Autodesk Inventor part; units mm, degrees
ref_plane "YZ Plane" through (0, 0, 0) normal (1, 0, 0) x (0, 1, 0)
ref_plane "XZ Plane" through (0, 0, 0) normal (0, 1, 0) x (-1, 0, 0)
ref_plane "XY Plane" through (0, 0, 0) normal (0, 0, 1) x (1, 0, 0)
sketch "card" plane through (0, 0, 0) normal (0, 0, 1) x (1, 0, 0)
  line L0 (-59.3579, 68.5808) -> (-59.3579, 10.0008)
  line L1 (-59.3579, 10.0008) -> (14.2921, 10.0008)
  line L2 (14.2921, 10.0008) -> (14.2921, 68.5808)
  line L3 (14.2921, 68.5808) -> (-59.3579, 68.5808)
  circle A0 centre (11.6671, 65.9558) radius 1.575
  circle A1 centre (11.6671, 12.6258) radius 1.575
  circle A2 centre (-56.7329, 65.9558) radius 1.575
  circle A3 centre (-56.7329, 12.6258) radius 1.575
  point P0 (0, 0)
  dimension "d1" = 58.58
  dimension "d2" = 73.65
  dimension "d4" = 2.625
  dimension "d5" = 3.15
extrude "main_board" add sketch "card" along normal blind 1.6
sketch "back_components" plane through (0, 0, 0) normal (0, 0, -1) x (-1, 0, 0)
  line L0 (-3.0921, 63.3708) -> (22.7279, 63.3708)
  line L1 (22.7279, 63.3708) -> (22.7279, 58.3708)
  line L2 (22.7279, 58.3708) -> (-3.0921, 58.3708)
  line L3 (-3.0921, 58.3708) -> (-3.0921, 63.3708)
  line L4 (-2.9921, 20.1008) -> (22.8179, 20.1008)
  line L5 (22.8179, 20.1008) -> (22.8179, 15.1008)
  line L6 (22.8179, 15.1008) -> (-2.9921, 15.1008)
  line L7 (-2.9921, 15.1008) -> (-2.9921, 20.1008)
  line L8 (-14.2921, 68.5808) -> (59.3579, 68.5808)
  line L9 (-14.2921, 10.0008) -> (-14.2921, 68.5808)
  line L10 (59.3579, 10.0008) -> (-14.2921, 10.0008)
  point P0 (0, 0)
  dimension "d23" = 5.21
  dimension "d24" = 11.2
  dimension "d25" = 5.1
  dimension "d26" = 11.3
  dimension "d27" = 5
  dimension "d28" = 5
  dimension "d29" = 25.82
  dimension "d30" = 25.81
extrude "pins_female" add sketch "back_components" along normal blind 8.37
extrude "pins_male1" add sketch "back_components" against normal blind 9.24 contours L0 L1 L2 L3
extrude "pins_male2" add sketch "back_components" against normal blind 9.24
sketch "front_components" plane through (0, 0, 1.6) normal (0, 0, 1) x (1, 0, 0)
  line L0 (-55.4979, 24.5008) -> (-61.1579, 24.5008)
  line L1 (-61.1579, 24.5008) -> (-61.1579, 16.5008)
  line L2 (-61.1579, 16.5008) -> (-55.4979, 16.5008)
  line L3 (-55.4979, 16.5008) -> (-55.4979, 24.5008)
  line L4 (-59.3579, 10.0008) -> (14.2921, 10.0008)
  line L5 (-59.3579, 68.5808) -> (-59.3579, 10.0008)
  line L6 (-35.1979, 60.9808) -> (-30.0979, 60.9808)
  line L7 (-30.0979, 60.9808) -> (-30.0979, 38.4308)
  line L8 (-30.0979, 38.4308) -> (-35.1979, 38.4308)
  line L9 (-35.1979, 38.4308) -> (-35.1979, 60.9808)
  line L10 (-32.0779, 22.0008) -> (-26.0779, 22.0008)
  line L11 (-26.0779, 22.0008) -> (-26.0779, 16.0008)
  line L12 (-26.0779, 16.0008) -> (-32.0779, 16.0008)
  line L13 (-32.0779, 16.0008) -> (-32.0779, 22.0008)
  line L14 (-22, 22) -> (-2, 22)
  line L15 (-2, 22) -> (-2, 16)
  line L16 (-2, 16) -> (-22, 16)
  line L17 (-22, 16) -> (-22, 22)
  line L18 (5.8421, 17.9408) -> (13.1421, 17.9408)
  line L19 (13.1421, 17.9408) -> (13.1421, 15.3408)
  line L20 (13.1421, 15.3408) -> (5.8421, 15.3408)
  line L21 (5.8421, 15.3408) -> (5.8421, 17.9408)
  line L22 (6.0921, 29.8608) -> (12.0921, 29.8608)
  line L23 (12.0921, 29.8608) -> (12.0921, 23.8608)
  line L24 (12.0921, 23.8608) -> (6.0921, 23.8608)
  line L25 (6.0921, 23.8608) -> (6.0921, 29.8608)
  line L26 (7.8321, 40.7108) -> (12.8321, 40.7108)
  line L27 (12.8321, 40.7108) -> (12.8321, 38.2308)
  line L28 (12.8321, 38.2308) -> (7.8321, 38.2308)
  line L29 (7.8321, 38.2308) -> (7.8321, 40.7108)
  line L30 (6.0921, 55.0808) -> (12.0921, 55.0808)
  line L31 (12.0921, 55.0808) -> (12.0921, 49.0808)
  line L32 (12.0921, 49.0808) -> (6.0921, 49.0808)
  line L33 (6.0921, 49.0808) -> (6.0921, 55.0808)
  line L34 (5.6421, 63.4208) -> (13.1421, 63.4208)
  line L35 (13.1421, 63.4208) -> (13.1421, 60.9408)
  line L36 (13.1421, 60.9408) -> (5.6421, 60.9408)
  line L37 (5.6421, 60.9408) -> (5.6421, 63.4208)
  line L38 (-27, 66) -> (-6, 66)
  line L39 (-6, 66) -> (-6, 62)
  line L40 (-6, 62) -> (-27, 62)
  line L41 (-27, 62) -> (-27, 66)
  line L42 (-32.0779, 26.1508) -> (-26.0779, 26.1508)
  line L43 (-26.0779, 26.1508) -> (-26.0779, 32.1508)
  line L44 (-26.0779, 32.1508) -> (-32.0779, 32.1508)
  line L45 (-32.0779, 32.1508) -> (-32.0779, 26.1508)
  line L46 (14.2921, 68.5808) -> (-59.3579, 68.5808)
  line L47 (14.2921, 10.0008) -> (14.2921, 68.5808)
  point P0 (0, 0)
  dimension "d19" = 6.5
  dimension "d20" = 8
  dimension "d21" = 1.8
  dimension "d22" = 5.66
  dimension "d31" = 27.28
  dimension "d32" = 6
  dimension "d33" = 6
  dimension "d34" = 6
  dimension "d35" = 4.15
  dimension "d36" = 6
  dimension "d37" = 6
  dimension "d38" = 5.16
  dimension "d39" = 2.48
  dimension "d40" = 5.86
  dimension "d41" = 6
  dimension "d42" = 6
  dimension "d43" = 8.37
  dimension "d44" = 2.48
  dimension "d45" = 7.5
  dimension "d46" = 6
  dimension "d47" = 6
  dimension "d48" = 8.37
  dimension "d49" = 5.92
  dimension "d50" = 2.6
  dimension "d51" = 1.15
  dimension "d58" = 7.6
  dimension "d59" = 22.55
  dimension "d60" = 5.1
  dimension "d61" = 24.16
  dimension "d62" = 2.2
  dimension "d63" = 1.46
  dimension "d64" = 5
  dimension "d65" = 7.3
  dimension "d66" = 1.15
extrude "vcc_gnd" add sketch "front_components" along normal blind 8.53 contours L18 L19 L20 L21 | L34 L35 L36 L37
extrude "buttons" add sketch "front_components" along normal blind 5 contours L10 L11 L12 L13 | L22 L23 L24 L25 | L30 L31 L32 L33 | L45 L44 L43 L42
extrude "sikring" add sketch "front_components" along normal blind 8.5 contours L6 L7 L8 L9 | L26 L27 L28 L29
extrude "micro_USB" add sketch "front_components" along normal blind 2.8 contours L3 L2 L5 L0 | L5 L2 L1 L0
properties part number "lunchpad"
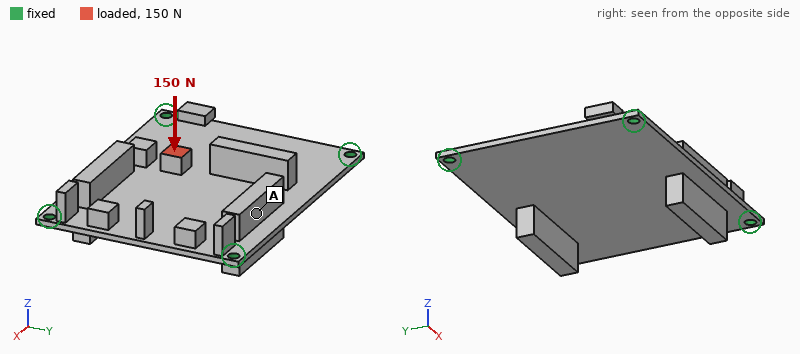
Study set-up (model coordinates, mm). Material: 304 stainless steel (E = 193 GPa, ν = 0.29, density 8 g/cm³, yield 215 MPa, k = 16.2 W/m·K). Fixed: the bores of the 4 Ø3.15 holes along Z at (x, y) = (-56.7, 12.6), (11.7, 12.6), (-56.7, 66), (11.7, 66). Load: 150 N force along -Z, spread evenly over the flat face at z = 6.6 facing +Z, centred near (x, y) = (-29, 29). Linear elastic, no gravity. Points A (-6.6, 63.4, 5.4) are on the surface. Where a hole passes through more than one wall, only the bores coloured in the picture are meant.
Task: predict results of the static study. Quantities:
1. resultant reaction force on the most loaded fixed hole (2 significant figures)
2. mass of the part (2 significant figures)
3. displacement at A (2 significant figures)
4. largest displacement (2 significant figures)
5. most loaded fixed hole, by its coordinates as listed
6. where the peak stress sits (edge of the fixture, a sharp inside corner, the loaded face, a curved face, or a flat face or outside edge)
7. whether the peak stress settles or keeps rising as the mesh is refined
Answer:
67 N
110 g
19 µm
87 µm
(-56.7, 12.6)
edge of the fixture
keeps rising
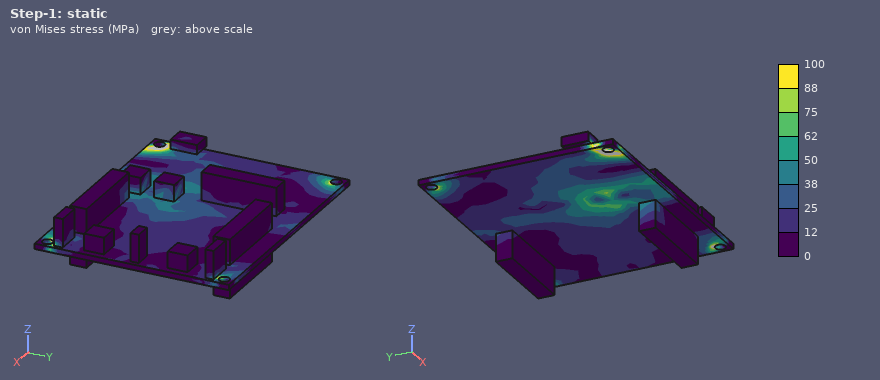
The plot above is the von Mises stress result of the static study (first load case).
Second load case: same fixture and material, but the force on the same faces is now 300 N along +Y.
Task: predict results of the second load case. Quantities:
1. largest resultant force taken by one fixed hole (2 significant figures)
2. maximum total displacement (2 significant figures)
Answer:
110 N
34 µm
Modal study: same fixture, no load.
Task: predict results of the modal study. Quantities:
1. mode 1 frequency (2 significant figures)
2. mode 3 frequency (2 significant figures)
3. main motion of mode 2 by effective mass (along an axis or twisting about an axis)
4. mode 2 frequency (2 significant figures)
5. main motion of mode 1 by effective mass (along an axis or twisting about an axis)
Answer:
1100 Hz
2500 Hz
twisting about X
1800 Hz
along Z
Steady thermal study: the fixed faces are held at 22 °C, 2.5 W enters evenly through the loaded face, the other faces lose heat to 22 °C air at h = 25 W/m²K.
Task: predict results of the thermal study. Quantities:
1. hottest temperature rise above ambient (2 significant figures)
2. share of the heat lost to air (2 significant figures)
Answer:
53 K
78 %
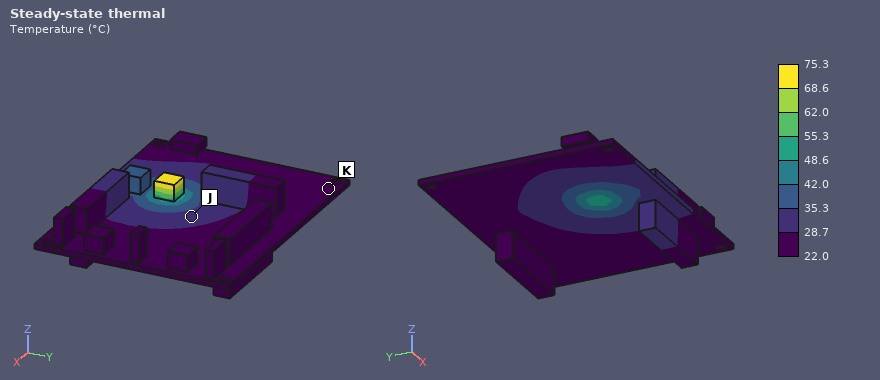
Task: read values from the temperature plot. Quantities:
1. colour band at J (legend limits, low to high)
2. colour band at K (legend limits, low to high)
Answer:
28.7 to 35.3 °C
22.0 to 28.7 °C
